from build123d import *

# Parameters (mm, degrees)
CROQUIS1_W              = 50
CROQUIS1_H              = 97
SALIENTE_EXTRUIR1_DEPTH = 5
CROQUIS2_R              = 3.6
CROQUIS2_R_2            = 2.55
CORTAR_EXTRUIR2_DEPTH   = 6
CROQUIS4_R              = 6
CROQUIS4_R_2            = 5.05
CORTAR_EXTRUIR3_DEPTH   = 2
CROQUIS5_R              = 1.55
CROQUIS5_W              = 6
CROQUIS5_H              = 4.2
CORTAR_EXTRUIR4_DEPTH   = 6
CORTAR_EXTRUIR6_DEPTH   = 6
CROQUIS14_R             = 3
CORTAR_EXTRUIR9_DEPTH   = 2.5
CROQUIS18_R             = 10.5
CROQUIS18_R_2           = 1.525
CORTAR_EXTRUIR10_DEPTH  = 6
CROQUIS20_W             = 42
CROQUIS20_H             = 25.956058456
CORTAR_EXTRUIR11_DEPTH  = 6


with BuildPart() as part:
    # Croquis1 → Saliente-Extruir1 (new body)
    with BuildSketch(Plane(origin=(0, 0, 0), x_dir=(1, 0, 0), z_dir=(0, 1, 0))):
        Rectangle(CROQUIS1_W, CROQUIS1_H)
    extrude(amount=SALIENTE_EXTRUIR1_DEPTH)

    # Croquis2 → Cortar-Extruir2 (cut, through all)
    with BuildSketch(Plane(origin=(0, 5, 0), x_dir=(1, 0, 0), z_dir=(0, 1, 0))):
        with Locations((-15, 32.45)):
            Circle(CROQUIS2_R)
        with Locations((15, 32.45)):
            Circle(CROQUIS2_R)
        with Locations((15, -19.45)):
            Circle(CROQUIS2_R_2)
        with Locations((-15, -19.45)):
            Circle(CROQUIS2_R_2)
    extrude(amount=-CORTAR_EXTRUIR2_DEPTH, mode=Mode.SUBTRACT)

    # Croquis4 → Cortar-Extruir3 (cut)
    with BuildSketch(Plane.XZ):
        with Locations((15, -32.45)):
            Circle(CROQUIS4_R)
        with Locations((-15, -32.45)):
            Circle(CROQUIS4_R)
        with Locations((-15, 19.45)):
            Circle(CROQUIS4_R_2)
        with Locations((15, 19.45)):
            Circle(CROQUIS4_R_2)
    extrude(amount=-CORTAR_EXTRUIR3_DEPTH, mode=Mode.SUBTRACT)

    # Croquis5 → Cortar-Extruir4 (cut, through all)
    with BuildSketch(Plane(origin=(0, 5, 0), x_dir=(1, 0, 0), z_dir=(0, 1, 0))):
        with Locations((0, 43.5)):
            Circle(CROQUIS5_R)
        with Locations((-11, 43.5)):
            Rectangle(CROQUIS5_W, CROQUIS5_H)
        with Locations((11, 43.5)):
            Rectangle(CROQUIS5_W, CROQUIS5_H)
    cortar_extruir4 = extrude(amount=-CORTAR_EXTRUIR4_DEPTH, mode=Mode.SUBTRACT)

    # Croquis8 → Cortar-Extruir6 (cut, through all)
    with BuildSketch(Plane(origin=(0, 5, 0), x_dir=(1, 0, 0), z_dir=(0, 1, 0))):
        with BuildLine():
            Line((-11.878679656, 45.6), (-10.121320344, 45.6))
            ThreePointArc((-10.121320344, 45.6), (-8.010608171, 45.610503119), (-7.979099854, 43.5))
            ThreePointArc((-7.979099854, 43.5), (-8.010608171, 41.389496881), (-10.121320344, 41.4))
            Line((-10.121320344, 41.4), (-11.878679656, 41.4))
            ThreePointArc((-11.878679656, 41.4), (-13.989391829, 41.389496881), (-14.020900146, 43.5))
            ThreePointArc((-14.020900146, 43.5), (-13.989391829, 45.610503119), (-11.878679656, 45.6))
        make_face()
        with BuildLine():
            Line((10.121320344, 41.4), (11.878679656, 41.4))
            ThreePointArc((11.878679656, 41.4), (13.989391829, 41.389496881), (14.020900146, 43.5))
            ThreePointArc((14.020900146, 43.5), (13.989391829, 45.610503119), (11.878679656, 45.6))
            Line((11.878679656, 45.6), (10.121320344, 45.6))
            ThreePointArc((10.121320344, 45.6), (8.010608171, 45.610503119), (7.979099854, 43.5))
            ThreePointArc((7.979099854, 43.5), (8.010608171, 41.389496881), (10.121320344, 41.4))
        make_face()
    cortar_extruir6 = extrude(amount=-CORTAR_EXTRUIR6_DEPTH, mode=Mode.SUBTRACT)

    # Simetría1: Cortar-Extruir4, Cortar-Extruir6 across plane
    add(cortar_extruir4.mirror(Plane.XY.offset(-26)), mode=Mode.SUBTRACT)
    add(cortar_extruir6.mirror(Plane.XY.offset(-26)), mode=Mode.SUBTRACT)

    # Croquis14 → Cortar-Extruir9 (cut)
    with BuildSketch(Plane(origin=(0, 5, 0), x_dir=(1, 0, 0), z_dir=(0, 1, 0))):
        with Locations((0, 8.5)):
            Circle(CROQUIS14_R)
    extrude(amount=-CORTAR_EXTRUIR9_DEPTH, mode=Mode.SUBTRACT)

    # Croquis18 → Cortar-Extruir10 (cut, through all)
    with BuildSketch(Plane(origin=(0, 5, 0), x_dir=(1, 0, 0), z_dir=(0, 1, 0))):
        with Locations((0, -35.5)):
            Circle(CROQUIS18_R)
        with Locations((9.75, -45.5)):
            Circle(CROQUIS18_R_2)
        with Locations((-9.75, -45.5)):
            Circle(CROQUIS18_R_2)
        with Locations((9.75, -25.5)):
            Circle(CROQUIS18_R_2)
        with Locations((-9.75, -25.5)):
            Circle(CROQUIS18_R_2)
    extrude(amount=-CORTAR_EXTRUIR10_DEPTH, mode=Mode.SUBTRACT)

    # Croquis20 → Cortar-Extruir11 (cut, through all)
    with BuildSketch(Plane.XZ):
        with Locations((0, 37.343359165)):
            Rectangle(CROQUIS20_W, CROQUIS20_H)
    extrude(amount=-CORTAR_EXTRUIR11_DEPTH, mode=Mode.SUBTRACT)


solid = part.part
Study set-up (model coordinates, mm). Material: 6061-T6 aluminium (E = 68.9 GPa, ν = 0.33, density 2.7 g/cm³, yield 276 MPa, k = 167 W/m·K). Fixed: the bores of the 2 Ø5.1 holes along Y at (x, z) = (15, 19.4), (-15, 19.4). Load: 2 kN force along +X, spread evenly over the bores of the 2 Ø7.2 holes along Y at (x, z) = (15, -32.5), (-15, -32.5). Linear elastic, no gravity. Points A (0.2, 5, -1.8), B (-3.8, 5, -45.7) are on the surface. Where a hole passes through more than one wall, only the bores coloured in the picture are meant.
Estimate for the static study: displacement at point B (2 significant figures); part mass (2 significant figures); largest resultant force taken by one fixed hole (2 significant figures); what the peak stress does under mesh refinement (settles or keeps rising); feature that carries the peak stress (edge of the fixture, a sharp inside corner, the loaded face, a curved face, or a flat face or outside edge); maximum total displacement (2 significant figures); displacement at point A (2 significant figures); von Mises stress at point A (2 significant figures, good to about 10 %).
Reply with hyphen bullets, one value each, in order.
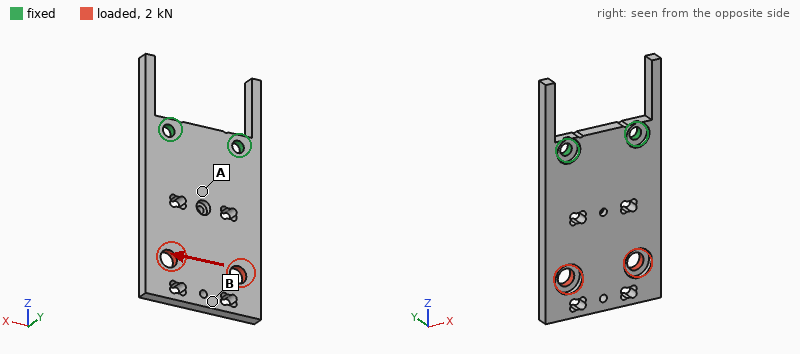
- 0.098 mm
- 47 g
- 3.3 kN
- keeps rising
- edge of the fixture
- 0.13 mm
- 0.026 mm
- 41 MPa
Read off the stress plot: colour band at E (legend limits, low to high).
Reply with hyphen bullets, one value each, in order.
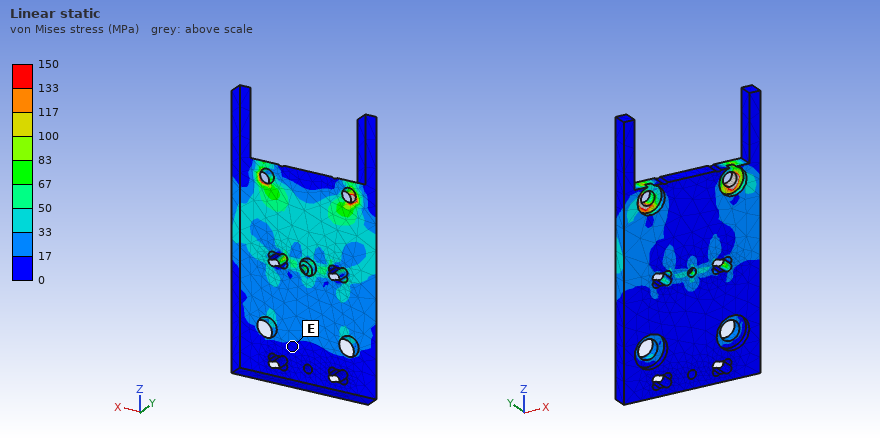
- 0 to 17 MPa
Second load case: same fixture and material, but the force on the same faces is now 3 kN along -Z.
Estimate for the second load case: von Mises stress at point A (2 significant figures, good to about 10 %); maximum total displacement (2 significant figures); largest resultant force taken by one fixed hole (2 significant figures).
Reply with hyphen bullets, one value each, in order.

- 19 MPa
- 0.18 mm
- 1.5 kN
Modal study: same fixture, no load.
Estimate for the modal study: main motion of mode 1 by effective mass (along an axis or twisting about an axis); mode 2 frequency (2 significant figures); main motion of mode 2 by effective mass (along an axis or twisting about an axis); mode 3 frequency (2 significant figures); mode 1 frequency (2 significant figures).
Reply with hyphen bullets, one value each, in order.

- along Y
- 2500 Hz
- twisting about Z
- 4200 Hz
- 780 Hz
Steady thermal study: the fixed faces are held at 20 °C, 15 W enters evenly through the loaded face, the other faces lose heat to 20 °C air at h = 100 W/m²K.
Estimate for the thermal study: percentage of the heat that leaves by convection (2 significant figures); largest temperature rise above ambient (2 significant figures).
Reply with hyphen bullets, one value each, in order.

- 47 %
- 16 K
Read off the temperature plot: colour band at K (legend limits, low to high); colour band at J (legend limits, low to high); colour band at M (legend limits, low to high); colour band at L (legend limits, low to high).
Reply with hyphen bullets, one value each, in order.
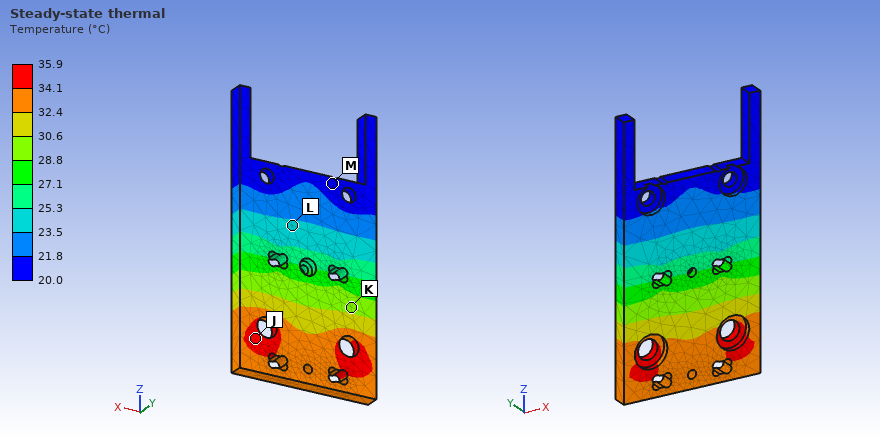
- 28.8 to 30.6 °C
- 34.1 to 35.9 °C
- 20.0 to 21.8 °C
- 23.5 to 25.3 °C
